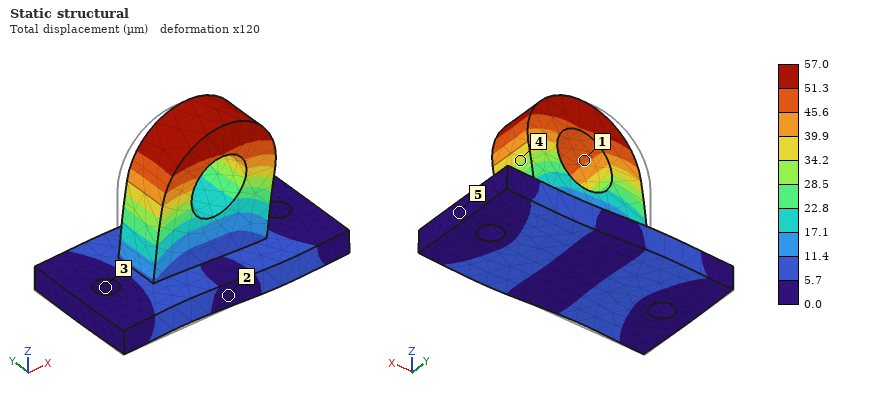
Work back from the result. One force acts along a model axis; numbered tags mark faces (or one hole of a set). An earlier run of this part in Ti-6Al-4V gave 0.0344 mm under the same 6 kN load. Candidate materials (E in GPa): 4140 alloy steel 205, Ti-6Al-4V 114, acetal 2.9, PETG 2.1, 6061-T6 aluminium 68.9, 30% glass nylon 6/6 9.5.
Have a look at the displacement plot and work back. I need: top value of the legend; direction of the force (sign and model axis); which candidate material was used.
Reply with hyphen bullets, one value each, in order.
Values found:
- 57.0 µm
- +X
- 6061-T6 aluminium
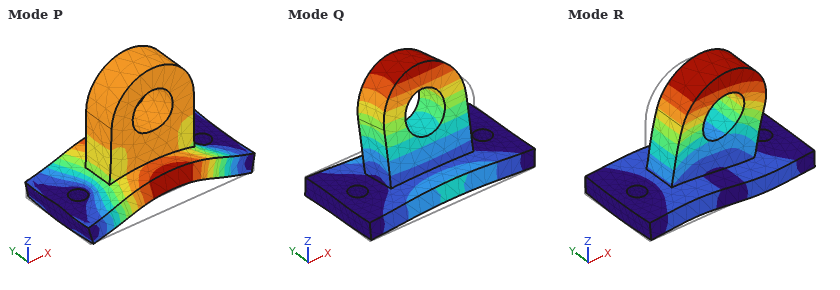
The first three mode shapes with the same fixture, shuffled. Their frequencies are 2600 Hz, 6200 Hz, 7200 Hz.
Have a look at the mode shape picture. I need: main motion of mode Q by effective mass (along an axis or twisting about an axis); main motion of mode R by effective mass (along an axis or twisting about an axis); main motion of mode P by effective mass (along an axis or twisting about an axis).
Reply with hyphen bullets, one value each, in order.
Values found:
- along Y
- along X
- along Z
